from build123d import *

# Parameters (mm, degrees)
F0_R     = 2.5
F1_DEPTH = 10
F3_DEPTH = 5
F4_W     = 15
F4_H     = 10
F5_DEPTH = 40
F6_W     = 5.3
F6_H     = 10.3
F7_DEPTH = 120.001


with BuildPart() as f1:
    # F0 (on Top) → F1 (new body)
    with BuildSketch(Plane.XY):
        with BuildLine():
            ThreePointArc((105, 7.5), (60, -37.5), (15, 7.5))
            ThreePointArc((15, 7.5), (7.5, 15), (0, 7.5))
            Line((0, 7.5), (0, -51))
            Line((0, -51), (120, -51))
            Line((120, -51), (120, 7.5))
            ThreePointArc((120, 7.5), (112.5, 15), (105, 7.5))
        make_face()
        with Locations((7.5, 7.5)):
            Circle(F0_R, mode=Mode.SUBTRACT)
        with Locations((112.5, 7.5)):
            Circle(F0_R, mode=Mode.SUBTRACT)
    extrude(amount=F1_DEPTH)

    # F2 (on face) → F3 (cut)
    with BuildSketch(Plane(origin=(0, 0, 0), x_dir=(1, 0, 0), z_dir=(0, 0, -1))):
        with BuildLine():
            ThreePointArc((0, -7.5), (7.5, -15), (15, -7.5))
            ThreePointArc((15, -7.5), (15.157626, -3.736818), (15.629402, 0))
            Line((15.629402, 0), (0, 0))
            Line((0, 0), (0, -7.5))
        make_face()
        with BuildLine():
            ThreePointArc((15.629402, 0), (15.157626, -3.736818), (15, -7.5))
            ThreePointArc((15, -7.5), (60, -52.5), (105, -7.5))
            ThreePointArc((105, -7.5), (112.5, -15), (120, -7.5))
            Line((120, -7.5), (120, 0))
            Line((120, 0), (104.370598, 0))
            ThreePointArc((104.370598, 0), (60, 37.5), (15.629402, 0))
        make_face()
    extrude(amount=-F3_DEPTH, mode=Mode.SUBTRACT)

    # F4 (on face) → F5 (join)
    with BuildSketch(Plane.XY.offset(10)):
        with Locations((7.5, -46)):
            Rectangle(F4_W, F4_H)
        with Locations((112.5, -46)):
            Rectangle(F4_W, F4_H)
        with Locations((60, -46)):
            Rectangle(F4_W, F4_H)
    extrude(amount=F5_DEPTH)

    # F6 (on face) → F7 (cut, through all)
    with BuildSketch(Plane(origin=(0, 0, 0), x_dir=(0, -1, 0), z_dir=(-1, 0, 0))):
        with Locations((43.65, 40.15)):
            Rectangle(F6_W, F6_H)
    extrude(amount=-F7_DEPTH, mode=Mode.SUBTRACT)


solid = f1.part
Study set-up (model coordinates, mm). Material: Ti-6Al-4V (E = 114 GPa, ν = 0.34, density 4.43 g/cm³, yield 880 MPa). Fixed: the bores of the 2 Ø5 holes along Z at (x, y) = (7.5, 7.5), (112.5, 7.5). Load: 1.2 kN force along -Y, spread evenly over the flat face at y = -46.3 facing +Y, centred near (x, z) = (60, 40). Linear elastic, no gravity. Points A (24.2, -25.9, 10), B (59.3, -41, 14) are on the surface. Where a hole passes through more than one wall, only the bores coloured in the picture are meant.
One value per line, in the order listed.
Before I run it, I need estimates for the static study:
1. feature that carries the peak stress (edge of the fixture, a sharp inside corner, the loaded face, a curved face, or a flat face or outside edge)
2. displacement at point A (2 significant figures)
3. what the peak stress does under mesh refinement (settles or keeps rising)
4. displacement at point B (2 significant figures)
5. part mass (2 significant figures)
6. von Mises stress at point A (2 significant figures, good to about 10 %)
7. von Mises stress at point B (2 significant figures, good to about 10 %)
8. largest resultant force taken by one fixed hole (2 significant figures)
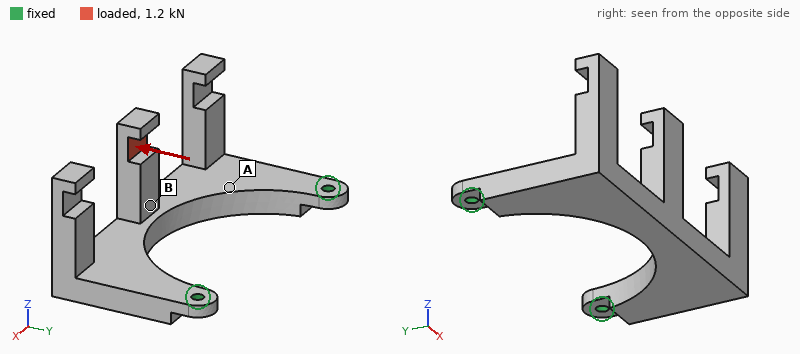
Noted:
edge of the fixture
0.29 mm
keeps rising
0.49 mm
240 g
57 MPa
120 MPa
790 N
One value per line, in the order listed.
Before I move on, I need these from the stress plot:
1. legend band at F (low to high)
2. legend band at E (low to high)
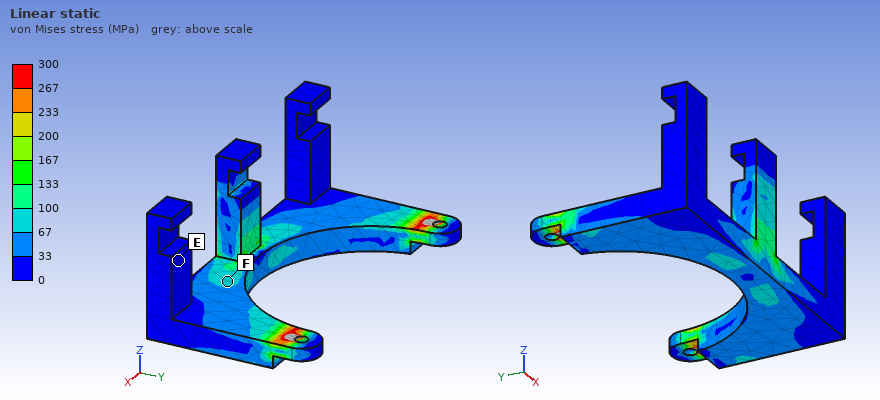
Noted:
67 to 100 MPa
0 to 33 MPa
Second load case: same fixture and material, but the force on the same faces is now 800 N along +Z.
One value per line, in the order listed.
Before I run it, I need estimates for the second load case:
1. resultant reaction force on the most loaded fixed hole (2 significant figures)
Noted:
400 N
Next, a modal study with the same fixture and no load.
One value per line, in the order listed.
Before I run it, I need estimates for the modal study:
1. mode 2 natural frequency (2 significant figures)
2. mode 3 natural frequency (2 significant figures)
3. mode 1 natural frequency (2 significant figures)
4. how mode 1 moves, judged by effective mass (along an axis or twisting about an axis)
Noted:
1100 Hz
2000 Hz
470 Hz
along Z
